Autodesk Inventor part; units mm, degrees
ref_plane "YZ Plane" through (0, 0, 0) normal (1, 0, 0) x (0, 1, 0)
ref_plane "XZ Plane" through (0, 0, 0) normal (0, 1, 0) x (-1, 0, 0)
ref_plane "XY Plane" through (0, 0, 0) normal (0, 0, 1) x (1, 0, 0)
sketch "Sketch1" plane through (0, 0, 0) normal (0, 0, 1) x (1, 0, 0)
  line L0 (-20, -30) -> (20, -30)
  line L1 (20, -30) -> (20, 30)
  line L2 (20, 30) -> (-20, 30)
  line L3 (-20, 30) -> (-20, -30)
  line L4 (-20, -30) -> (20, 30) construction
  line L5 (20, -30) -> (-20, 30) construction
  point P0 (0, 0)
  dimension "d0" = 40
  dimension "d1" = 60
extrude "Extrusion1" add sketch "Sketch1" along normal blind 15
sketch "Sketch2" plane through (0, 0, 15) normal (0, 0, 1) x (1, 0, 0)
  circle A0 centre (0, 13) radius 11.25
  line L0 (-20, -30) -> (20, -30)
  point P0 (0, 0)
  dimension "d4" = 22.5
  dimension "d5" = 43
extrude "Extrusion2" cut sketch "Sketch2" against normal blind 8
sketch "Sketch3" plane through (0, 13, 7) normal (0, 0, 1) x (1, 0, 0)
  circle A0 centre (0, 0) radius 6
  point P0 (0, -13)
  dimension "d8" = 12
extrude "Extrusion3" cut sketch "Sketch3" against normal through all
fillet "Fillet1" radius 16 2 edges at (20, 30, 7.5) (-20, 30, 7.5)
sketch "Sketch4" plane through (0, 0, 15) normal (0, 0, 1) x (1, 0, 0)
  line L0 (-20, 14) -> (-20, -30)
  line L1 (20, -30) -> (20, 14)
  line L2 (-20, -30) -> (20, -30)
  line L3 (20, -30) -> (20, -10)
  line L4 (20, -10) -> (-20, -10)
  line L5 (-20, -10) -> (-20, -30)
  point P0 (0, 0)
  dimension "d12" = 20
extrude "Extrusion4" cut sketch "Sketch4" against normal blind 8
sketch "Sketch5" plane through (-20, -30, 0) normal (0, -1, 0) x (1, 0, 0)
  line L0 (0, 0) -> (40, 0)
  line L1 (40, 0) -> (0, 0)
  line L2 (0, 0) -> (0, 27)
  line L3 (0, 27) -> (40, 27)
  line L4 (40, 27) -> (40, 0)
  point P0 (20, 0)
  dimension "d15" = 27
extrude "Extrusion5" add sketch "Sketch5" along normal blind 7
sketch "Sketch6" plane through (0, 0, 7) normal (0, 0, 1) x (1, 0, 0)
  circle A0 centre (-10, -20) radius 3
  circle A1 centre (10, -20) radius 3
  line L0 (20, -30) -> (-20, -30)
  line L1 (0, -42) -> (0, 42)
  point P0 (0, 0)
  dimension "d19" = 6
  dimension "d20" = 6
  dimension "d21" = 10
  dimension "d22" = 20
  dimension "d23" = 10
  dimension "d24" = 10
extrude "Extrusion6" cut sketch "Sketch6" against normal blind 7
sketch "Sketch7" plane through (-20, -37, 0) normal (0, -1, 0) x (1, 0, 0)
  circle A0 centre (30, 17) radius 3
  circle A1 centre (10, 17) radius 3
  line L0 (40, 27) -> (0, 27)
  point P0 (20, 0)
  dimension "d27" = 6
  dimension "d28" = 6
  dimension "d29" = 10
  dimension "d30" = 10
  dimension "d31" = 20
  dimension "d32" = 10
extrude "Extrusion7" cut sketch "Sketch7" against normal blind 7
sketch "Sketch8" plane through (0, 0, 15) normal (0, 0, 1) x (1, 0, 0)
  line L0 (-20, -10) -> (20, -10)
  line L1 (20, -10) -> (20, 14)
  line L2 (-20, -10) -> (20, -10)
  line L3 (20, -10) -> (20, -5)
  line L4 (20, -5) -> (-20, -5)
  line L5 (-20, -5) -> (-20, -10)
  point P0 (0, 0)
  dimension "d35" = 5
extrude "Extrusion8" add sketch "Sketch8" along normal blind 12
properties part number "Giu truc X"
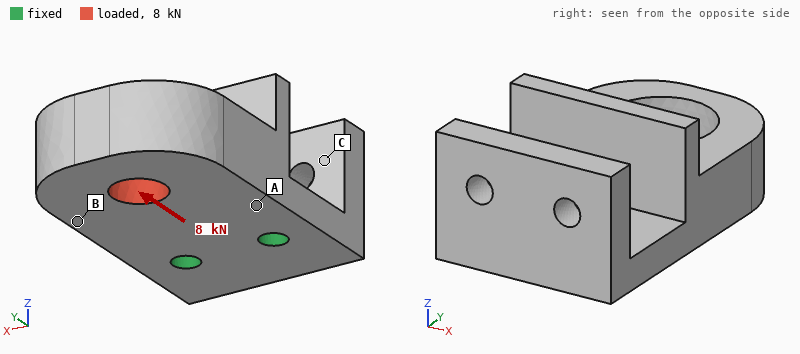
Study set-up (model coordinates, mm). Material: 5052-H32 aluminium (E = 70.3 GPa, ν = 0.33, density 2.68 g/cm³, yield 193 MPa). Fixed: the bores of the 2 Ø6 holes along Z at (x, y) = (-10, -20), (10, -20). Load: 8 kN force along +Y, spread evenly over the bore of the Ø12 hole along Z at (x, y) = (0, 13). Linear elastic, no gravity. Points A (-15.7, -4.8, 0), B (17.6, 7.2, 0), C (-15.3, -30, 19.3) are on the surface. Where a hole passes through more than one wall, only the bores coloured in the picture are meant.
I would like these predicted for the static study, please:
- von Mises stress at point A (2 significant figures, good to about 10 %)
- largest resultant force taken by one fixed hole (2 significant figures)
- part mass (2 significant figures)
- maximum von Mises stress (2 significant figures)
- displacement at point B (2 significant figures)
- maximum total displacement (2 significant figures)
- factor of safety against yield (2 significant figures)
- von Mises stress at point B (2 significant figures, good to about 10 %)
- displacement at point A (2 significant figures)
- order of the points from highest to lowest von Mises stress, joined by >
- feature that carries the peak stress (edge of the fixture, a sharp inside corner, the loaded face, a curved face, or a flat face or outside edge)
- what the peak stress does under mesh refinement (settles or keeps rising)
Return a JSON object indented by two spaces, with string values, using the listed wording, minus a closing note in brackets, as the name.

{
  "von Mises stress at point A": "33 MPa",
  "largest resultant force taken by one fixed hole": "4.0 kN",
  "part mass": "89 g",
  "maximum von Mises stress": "81 MPa",
  "displacement at point B": "13 µm",
  "maximum total displacement": "33 µm",
  "factor of safety against yield": "2.4",
  "von Mises stress at point B": "20 MPa",
  "displacement at point A": "7.7 µm",
  "order of the points from highest to lowest von Mises stress, joined by >": "A > B > C",
  "feature that carries the peak stress": "the loaded face",
  "what the peak stress does under mesh refinement": "settles"
}
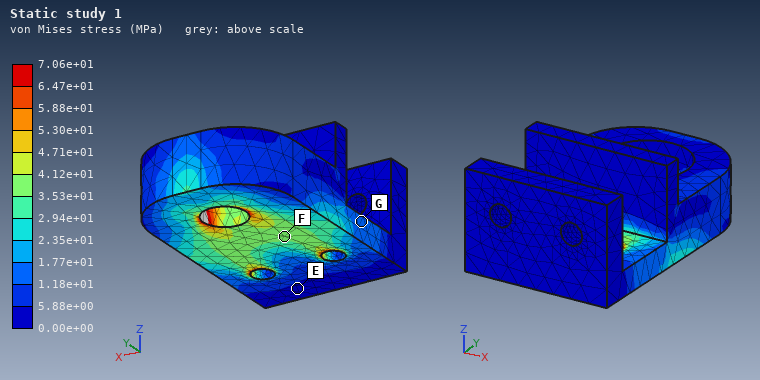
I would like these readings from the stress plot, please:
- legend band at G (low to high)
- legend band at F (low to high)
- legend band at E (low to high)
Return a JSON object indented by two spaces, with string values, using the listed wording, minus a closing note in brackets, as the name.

{
  "legend band at G": "1.18e+01 to 1.77e+01 MPa",
  "legend band at F": "3.53e+01 to 4.12e+01 MPa",
  "legend band at E": "0.00e+00 to 5.88e+00 MPa"
}
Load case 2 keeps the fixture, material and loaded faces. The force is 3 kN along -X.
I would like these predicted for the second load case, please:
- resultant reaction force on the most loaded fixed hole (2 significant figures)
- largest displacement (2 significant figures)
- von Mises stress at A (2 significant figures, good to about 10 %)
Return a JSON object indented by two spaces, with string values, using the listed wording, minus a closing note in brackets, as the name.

{
  "resultant reaction force on the most loaded fixed hole": "4.3 kN",
  "largest displacement": "49 µm",
  "von Mises stress at A": "24 MPa"
}
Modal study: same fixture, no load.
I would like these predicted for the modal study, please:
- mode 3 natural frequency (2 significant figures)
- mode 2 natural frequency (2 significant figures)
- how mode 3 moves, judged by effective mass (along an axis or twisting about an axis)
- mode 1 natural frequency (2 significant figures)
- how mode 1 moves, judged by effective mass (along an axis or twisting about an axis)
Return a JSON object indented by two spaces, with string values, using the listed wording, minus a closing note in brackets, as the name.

{
  "mode 3 natural frequency": "7000 Hz",
  "mode 2 natural frequency": "5900 Hz",
  "how mode 3 moves, judged by effective mass": "along X",
  "mode 1 natural frequency": "2200 Hz",
  "how mode 1 moves, judged by effective mass": "along Z"
}
